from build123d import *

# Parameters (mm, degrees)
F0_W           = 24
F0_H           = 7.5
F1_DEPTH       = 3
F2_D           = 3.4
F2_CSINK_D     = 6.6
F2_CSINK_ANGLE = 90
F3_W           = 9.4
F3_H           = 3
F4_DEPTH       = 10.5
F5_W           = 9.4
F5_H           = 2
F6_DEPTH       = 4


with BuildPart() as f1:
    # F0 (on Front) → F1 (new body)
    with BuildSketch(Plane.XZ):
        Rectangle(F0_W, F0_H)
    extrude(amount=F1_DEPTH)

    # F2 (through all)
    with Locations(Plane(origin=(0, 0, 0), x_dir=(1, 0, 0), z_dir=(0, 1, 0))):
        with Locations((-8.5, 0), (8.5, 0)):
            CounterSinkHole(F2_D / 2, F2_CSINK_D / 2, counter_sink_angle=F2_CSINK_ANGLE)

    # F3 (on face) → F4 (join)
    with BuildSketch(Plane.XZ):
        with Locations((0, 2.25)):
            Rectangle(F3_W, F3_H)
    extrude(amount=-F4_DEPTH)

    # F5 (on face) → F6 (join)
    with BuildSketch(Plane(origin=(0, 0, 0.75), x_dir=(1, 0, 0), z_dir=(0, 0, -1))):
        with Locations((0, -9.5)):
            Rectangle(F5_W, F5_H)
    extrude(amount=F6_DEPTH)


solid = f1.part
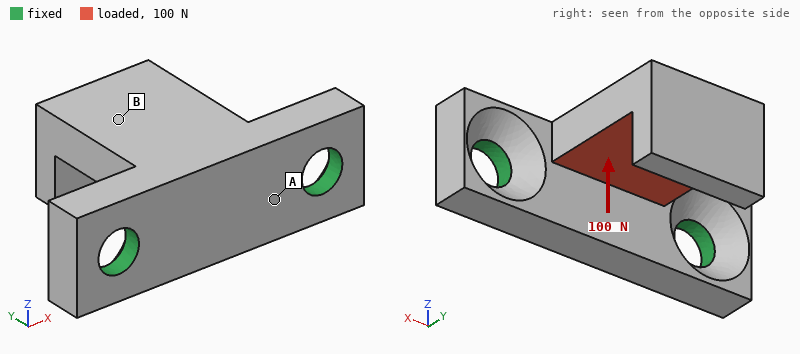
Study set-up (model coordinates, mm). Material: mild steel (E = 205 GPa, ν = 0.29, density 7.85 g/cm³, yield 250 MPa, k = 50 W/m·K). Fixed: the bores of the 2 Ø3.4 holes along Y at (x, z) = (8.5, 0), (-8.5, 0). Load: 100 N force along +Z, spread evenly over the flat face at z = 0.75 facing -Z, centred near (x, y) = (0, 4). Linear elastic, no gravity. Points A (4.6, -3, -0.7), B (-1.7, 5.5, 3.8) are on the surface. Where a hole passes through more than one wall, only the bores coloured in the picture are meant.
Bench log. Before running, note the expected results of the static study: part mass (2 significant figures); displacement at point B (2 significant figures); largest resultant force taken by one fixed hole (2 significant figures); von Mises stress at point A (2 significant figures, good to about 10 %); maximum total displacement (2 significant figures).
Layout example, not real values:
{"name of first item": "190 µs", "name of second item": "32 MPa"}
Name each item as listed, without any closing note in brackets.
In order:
{"part mass": "6.4 g", "displacement at point B": "6.4 µm", "largest resultant force taken by one fixed hole": "50 N", "von Mises stress at point A": "15 MPa", "maximum total displacement": "11 µm"}
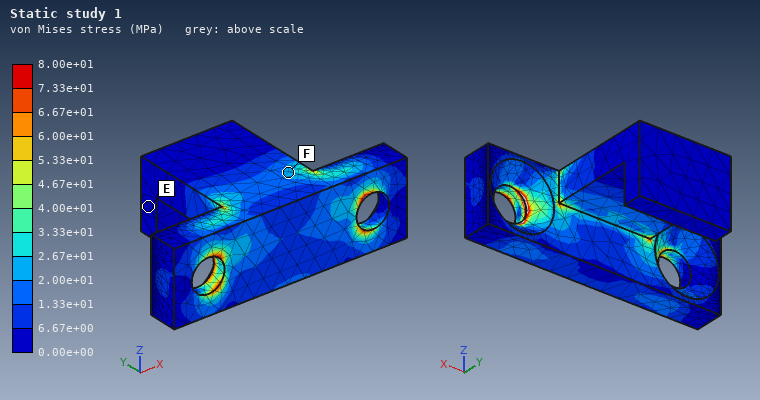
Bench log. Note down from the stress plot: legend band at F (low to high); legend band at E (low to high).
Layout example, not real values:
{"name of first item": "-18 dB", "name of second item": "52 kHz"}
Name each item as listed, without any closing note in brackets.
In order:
{"legend band at F": "2.00e+01 to 2.67e+01 MPa", "legend band at E": "0.00e+00 to 6.67e+00 MPa"}
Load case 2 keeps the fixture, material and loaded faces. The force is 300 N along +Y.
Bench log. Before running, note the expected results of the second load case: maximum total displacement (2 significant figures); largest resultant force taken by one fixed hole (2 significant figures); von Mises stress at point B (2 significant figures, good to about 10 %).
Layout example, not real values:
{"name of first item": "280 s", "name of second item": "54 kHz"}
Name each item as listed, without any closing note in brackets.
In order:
{"maximum total displacement": "5.3 µm", "largest resultant force taken by one fixed hole": "190 N", "von Mises stress at point B": "7.6 MPa"}
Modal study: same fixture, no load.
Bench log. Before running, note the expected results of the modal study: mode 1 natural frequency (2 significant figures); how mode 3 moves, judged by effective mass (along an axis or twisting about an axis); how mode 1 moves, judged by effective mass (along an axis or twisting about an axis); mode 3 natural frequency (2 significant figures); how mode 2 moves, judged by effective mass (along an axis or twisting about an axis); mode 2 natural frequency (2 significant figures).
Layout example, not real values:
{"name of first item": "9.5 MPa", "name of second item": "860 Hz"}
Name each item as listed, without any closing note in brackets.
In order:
{"mode 1 natural frequency": "8600 Hz", "how mode 3 moves, judged by effective mass": "along Y", "how mode 1 moves, judged by effective mass": "along Z", "mode 3 natural frequency": "29 kHz", "how mode 2 moves, judged by effective mass": "along X", "mode 2 natural frequency": "20 kHz"}
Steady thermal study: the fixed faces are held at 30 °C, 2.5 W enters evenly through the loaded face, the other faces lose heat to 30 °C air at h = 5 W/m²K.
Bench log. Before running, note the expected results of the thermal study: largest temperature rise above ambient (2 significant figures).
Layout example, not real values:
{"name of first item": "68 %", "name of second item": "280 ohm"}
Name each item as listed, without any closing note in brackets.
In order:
{"largest temperature rise above ambient": "16 K"}
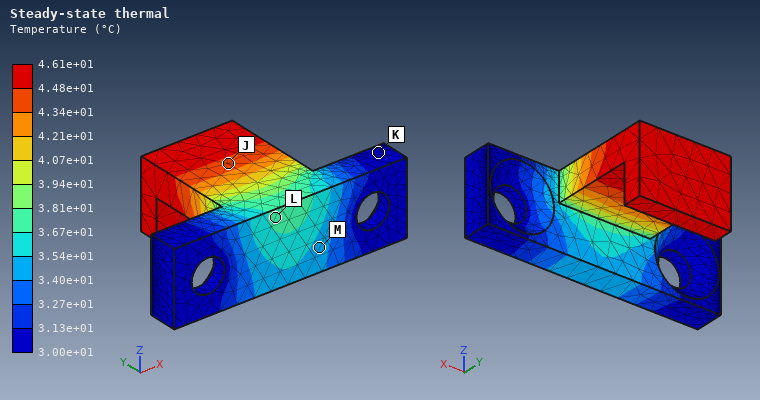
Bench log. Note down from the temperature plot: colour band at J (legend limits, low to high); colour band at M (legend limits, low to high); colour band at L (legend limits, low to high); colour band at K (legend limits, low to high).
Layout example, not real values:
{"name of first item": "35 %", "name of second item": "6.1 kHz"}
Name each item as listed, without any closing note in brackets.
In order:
{"colour band at J": "4.34e+01 to 4.48e+01 °C", "colour band at M": "3.40e+01 to 3.54e+01 °C", "colour band at L": "3.67e+01 to 3.81e+01 °C", "colour band at K": "3.00e+01 to 3.13e+01 °C"}
